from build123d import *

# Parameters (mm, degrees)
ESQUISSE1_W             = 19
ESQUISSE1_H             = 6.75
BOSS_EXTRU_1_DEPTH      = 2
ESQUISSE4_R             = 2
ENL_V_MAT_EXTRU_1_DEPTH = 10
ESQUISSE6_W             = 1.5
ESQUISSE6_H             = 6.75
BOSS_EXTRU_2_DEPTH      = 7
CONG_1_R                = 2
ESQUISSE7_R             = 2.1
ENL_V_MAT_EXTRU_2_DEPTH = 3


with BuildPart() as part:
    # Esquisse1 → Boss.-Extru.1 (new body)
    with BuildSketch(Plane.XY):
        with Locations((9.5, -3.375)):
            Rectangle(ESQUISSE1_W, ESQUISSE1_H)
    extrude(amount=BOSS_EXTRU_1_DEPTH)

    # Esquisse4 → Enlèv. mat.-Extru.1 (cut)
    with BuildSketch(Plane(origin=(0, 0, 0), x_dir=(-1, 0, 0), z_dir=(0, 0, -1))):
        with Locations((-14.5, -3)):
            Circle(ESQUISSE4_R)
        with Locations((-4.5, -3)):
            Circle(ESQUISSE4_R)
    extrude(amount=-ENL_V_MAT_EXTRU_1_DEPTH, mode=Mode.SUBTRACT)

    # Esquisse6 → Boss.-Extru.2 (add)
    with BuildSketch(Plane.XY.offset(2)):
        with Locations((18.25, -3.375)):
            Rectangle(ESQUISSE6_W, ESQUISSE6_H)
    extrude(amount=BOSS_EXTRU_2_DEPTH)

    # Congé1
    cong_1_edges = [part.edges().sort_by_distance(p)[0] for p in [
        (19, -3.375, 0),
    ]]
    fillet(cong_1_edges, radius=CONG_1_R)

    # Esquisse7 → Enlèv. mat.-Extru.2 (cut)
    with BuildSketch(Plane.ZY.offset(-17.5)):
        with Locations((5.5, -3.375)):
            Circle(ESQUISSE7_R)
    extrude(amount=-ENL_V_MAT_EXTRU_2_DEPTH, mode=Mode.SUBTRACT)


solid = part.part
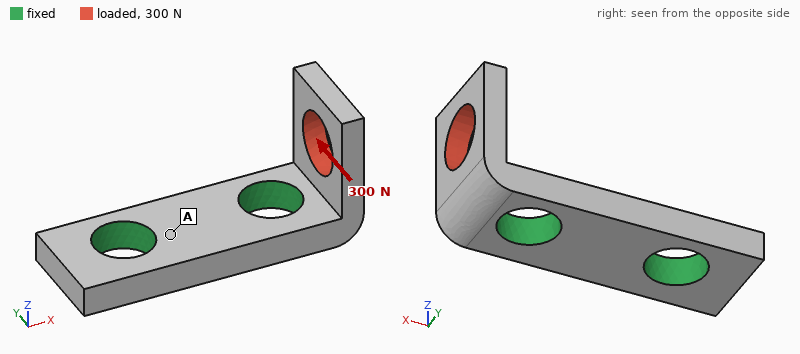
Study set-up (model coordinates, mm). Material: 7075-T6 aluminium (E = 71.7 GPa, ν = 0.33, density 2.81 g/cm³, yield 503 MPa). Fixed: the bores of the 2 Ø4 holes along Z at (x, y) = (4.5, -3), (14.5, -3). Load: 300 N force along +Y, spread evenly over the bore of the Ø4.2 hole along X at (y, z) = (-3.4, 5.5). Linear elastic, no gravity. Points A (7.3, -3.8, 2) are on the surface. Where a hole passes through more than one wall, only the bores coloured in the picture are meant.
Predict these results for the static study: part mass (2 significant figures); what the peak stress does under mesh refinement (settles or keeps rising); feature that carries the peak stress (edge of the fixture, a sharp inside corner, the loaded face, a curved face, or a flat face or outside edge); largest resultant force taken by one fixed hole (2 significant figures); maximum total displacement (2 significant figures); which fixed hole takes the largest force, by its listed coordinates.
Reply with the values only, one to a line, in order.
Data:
0.70 g
keeps rising
edge of the fixture
310 N
79 µm
(14.5, -3)
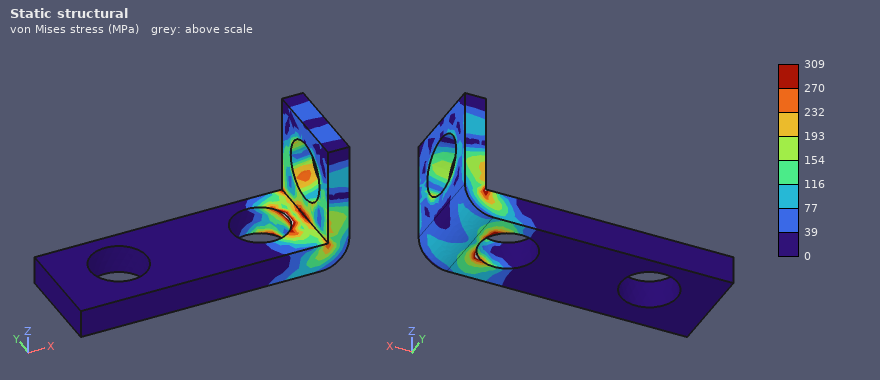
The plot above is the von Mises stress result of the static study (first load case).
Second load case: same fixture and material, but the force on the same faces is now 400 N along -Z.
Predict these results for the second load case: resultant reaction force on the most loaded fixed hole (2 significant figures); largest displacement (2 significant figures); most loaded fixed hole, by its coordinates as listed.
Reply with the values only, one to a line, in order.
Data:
400 N
37 µm
(14.5, -3)
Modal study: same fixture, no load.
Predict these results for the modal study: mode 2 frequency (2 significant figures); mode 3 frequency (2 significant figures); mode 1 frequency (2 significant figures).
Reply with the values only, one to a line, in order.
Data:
29 kHz
38 kHz
16 kHz
